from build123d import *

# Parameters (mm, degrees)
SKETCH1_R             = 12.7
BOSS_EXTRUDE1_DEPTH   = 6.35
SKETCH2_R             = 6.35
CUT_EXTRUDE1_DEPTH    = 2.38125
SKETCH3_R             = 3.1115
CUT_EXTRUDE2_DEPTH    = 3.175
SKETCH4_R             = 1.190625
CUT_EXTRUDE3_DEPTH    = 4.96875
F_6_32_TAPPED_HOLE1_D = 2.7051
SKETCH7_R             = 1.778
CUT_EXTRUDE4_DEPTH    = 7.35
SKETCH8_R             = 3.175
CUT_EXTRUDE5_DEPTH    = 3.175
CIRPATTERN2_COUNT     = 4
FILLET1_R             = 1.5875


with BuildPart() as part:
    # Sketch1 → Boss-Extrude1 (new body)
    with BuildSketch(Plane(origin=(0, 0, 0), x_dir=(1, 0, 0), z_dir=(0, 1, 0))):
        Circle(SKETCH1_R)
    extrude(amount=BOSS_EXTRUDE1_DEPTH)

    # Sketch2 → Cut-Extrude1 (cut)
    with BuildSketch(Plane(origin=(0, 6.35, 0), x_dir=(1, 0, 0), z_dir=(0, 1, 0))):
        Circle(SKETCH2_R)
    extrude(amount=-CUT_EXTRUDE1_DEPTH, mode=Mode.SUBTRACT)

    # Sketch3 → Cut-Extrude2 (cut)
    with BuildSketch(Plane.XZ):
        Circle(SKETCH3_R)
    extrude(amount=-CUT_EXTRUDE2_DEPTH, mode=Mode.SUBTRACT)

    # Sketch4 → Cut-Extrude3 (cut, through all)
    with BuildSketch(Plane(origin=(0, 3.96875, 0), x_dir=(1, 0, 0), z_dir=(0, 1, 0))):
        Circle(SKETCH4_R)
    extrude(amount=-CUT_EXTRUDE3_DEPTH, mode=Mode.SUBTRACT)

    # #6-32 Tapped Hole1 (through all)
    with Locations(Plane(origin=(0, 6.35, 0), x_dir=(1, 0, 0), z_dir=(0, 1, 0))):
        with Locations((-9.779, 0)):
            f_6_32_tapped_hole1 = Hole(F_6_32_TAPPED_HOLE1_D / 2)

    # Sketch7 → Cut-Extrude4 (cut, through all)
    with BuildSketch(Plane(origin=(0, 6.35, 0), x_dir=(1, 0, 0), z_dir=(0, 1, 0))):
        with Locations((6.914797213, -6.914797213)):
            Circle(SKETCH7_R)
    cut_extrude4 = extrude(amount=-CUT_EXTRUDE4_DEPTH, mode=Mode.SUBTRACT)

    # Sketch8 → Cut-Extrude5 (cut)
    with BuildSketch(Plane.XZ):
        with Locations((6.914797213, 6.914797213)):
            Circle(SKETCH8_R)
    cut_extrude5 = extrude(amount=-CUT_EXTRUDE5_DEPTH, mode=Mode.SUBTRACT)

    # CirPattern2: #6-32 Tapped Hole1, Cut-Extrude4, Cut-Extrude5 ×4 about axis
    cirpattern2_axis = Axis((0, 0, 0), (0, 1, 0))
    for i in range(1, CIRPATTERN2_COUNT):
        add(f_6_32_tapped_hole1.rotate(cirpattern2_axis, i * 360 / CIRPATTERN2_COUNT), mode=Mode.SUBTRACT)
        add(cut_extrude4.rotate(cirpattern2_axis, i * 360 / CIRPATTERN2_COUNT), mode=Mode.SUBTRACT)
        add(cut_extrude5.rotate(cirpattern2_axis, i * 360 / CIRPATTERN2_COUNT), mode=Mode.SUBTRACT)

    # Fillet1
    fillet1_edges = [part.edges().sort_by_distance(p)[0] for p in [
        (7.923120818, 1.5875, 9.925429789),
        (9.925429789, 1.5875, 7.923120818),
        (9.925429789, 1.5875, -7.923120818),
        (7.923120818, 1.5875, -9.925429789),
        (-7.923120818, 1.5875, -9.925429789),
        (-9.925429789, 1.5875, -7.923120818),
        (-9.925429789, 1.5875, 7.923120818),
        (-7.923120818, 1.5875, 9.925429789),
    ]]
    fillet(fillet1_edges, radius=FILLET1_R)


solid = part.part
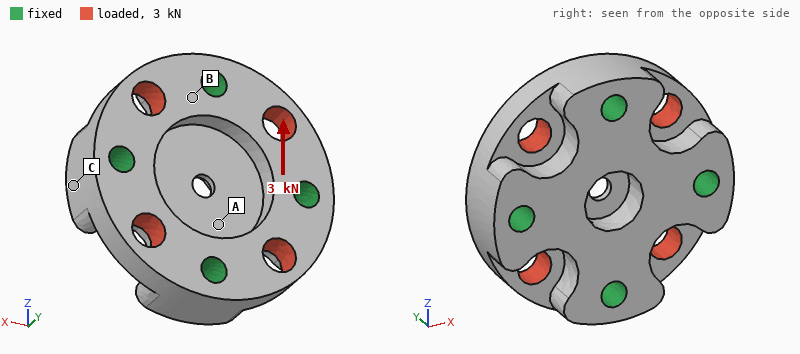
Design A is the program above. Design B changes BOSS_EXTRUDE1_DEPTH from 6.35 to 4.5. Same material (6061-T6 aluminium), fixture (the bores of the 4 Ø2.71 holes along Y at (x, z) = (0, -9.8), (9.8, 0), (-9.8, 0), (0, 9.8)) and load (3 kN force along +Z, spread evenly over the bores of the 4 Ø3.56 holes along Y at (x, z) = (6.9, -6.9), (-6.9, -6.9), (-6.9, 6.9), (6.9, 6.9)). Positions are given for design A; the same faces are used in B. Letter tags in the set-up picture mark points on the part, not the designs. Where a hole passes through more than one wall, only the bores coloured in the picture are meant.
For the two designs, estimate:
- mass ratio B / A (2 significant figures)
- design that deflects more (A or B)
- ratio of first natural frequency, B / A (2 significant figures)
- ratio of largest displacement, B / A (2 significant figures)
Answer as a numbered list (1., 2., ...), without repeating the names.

1. 0.72
2. B
3. 0.87
4. 2.0
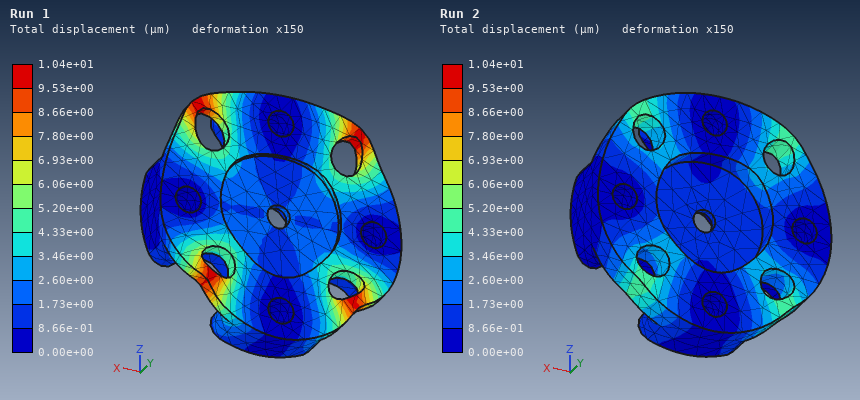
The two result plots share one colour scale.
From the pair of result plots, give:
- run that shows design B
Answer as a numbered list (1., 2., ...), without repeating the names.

1. Run 1
